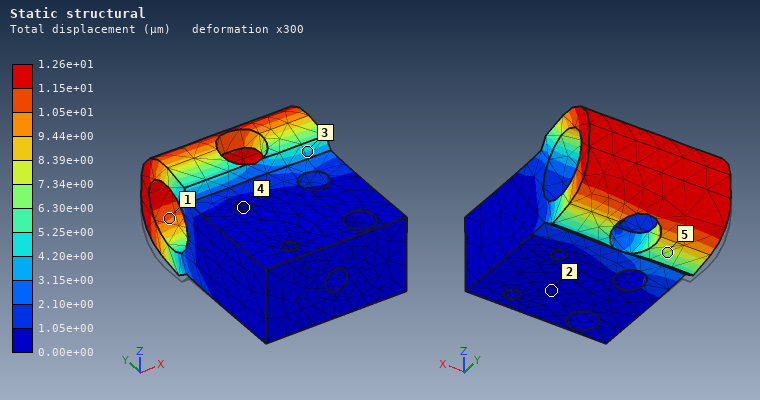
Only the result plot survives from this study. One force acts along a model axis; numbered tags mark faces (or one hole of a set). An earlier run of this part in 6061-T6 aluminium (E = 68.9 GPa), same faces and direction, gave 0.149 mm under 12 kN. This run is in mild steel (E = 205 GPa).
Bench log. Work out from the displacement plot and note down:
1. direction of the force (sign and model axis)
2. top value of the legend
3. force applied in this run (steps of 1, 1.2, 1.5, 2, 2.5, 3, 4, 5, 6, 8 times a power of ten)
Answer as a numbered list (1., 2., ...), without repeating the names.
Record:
1. +Z
2. 1.26e+01 µm
3. 3 kN
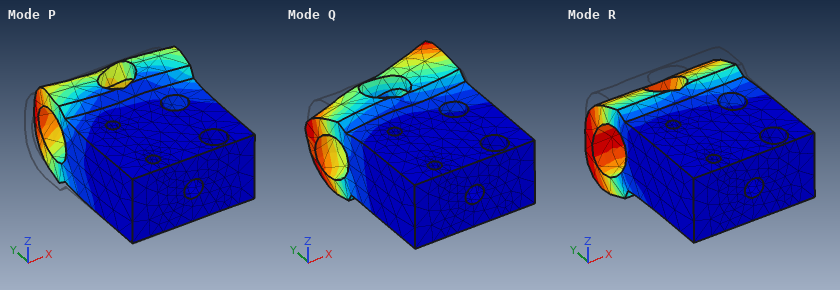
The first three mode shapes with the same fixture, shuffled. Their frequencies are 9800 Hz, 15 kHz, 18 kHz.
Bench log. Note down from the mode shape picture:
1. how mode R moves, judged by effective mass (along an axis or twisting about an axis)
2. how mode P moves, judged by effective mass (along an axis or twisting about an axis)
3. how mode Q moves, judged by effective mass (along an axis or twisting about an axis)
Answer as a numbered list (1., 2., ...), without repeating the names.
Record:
1. along Z
2. along X
3. twisting about Y
